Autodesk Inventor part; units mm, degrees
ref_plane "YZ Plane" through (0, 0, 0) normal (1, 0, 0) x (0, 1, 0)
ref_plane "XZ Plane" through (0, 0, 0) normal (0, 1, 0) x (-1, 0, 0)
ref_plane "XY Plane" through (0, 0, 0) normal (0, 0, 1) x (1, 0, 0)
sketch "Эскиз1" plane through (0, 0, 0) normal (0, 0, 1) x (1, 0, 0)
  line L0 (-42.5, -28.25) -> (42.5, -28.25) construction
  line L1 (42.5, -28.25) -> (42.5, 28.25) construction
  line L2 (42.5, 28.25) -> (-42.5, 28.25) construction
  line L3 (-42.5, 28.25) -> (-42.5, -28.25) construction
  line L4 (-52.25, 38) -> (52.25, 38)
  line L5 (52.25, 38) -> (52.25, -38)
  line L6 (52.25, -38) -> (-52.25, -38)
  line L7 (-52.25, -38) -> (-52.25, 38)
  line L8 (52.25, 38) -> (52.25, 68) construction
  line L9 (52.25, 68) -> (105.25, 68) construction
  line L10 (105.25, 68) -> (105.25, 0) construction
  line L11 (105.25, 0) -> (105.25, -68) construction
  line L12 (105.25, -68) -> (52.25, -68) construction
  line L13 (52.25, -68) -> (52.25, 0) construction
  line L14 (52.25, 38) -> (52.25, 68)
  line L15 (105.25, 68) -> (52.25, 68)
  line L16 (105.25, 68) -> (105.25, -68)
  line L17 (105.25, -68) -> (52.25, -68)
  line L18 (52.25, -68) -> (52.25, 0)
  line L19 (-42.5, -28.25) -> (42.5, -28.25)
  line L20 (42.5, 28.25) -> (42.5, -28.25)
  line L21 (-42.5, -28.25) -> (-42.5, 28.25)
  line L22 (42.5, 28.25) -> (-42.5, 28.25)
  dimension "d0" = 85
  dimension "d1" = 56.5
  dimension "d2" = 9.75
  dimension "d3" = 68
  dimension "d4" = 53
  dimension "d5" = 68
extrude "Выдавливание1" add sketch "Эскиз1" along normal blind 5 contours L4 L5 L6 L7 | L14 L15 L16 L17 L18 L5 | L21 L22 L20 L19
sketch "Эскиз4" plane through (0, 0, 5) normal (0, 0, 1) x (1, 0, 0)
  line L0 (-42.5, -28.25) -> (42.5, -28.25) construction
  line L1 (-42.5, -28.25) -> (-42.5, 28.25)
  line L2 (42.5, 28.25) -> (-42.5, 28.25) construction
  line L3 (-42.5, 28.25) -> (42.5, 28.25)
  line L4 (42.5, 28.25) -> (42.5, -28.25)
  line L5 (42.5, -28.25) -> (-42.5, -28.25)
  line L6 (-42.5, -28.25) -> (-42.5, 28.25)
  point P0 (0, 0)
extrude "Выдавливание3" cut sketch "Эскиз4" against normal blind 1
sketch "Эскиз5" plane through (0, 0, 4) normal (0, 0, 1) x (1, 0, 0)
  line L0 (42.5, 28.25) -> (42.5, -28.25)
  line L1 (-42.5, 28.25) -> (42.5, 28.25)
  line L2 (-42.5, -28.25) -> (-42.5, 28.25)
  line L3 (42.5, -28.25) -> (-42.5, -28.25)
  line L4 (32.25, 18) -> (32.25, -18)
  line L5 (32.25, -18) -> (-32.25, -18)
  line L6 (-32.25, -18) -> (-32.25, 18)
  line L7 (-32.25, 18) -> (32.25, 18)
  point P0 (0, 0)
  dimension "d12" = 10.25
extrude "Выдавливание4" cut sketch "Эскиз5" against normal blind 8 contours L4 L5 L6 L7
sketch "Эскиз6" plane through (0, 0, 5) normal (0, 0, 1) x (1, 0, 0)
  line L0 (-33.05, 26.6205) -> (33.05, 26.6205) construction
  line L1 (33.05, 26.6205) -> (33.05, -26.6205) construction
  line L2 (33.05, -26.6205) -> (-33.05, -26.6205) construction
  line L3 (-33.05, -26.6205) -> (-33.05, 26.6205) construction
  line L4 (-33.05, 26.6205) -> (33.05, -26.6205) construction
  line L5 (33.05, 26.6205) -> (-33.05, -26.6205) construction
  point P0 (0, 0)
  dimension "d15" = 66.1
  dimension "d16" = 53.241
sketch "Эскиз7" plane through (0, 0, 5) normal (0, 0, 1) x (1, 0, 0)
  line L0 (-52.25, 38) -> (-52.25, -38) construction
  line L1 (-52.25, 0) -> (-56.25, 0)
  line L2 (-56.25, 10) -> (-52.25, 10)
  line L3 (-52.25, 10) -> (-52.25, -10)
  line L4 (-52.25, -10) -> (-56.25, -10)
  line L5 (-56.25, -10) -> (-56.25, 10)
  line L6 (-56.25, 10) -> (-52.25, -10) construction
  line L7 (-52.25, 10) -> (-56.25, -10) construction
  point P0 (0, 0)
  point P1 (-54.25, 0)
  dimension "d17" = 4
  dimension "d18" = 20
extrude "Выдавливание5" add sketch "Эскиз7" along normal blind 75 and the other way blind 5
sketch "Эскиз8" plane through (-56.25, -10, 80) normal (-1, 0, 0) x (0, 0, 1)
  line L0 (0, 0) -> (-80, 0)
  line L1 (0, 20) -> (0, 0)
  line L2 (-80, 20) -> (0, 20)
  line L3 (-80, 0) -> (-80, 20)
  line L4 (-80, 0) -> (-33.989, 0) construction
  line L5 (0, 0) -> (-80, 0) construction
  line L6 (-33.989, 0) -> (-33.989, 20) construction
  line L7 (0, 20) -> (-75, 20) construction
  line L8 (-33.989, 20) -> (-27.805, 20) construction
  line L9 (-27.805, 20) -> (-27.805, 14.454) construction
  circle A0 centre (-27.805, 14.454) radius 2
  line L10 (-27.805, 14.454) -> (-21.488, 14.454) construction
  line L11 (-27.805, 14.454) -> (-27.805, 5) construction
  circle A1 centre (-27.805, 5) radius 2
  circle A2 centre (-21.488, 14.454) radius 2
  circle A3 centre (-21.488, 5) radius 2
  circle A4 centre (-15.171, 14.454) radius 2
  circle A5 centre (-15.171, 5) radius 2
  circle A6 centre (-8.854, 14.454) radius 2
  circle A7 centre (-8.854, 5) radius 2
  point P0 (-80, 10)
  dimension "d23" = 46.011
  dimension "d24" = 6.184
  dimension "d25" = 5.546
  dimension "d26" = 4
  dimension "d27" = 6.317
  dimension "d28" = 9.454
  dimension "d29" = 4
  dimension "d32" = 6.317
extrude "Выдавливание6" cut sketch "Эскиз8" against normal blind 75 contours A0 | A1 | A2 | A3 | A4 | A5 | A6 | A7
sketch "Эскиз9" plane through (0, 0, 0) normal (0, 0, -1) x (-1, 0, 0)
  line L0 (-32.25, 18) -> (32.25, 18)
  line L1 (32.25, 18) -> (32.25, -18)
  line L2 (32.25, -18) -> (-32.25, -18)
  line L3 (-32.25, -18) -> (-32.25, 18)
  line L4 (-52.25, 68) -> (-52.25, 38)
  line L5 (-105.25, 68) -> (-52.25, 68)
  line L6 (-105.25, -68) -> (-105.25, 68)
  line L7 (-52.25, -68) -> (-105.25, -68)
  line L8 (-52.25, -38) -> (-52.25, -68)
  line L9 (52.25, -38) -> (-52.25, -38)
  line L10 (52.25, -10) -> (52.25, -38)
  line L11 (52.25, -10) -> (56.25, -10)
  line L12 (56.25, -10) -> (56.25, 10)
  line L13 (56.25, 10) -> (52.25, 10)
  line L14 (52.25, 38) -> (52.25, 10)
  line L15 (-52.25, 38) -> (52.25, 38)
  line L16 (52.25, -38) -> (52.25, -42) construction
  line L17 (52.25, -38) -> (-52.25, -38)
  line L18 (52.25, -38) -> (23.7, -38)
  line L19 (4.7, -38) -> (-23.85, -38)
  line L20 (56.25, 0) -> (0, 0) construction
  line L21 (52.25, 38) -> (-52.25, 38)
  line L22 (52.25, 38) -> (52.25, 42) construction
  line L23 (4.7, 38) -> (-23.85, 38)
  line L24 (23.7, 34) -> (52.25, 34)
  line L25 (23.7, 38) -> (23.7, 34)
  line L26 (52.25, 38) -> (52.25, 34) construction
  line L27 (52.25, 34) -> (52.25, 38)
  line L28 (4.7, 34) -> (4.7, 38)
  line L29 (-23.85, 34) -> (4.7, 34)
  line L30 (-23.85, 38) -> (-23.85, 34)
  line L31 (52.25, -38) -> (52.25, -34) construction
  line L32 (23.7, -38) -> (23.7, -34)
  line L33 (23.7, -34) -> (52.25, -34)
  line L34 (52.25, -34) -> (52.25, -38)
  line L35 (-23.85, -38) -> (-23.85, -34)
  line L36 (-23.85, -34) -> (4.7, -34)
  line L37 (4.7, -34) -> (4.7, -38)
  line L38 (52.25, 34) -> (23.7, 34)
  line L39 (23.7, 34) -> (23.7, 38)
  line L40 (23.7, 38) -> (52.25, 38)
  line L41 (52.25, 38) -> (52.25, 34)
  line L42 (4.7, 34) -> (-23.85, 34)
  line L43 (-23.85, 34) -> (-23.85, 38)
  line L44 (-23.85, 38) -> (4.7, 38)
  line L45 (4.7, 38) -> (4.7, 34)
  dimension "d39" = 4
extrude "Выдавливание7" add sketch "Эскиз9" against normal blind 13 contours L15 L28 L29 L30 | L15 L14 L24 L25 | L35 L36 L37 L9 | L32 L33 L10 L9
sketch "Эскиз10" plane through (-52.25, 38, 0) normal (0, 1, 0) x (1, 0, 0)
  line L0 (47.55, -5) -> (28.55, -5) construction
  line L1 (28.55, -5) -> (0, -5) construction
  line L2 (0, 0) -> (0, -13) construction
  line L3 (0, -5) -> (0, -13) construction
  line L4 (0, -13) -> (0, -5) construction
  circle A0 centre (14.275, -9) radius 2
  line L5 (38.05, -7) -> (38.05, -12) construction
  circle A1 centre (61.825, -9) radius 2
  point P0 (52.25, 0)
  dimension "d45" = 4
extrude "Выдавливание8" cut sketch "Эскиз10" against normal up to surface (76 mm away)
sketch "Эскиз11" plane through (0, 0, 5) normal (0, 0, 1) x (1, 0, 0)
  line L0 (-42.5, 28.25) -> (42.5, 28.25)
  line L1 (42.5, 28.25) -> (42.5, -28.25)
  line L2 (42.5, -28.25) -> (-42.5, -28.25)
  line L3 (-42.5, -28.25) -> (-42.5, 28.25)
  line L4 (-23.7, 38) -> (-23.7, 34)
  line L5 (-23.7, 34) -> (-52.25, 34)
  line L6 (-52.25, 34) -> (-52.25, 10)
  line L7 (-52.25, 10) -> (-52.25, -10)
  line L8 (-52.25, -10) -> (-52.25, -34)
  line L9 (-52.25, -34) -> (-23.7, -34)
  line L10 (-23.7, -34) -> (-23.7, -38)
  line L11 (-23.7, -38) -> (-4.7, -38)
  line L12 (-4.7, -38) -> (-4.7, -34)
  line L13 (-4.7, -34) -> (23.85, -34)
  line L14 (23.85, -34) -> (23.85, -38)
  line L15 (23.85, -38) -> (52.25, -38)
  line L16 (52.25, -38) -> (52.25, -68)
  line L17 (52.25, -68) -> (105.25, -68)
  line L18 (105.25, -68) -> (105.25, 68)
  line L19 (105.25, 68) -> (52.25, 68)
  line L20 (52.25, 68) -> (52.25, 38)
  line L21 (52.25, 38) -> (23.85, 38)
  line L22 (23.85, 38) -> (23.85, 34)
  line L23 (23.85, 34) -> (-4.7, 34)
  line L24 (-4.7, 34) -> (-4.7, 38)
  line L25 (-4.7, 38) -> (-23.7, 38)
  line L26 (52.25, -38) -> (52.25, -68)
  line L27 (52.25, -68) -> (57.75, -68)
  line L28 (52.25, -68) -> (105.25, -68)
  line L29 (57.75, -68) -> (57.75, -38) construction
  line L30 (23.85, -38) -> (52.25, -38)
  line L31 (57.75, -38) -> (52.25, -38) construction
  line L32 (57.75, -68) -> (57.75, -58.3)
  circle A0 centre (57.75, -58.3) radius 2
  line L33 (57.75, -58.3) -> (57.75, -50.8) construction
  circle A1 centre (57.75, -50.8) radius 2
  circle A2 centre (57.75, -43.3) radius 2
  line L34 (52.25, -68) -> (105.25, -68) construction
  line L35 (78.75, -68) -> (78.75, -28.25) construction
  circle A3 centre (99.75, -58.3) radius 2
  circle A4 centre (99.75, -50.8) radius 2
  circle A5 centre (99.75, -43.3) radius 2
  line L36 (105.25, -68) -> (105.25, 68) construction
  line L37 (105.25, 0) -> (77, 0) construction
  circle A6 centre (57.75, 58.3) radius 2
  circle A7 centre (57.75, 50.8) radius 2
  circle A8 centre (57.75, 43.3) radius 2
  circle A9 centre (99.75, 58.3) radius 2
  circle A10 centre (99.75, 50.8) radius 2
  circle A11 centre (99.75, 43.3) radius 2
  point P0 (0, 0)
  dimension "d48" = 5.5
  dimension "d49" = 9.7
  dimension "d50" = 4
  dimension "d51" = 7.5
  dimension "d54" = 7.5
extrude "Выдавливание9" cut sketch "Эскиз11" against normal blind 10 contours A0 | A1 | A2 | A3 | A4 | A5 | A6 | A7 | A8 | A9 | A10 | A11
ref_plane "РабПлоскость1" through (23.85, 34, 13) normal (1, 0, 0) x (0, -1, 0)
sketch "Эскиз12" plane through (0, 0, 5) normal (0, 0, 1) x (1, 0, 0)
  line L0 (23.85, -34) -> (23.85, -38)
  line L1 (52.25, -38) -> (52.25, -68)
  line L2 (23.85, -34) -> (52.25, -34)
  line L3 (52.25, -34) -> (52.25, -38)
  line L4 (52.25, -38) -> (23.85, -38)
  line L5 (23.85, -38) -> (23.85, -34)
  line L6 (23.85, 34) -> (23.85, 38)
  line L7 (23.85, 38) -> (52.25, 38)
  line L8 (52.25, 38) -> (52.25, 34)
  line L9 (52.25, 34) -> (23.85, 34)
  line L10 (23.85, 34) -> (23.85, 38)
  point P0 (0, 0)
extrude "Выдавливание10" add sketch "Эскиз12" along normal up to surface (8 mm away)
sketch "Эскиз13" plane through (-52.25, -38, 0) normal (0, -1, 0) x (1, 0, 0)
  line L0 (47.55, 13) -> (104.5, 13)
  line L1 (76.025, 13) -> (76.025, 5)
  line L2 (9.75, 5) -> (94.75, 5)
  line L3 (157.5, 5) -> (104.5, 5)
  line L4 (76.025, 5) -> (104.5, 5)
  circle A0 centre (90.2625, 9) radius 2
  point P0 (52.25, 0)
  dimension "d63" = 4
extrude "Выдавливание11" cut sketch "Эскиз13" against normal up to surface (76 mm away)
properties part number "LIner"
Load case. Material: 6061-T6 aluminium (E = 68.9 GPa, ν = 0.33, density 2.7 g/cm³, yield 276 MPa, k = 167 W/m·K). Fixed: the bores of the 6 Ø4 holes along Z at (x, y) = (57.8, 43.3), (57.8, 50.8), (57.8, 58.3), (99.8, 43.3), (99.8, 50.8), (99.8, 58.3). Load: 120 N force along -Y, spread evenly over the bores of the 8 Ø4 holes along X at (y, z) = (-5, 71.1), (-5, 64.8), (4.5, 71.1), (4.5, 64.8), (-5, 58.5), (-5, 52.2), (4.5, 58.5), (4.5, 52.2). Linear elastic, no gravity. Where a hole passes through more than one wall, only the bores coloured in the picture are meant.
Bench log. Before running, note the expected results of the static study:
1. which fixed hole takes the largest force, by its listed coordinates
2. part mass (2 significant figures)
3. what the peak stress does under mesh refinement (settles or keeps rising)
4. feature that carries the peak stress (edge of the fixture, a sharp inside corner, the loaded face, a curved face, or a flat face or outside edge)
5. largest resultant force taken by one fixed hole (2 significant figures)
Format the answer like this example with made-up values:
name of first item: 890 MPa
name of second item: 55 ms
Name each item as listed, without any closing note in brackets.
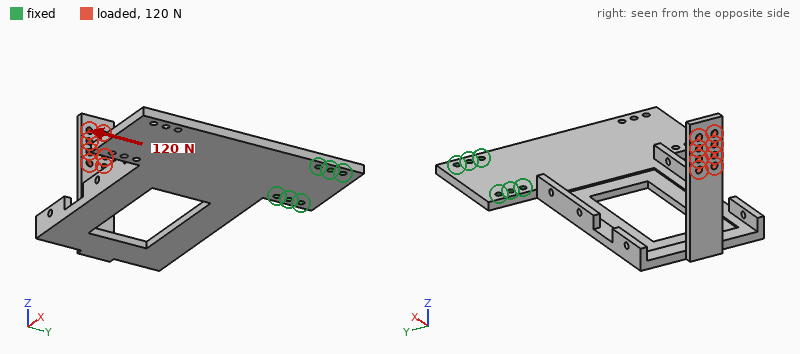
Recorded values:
which fixed hole takes the largest force, by its listed coordinates: (57.8, 43.3)
part mass: 190 g
what the peak stress does under mesh refinement: keeps rising
feature that carries the peak stress: edge of the fixture
largest resultant force taken by one fixed hole: 410 N
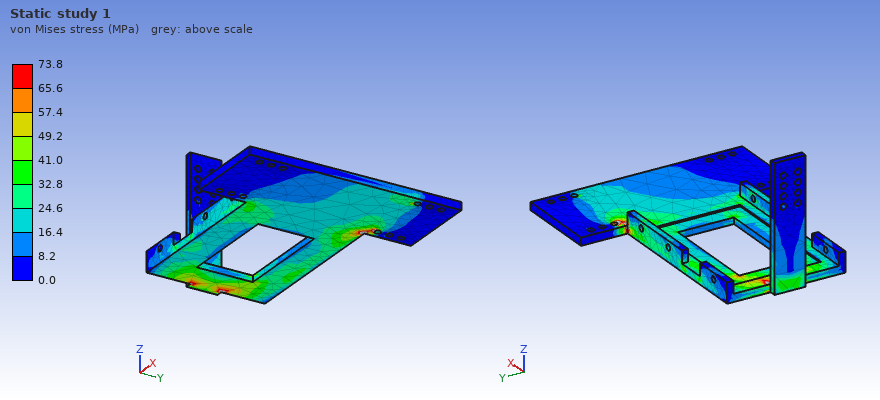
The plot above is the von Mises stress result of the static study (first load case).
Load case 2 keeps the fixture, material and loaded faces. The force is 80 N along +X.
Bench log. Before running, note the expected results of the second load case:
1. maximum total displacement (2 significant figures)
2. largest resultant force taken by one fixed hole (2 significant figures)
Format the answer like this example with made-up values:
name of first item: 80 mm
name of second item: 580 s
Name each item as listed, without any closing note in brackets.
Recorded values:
maximum total displacement: 2.4 mm
largest resultant force taken by one fixed hole: 150 N
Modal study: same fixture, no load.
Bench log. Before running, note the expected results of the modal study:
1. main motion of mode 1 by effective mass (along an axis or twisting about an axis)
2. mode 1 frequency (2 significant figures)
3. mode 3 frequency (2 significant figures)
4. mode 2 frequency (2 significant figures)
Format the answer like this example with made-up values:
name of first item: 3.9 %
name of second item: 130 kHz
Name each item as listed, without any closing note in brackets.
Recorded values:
main motion of mode 1 by effective mass: along Z
mode 1 frequency: 190 Hz
mode 3 frequency: 490 Hz
mode 2 frequency: 290 Hz
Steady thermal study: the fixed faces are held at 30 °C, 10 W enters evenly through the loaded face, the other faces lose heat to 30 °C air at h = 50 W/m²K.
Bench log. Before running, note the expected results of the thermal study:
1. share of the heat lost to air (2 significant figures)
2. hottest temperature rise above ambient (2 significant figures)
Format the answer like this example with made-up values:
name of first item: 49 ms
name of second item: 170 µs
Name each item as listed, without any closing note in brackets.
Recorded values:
share of the heat lost to air: 88 %
hottest temperature rise above ambient: 41 K
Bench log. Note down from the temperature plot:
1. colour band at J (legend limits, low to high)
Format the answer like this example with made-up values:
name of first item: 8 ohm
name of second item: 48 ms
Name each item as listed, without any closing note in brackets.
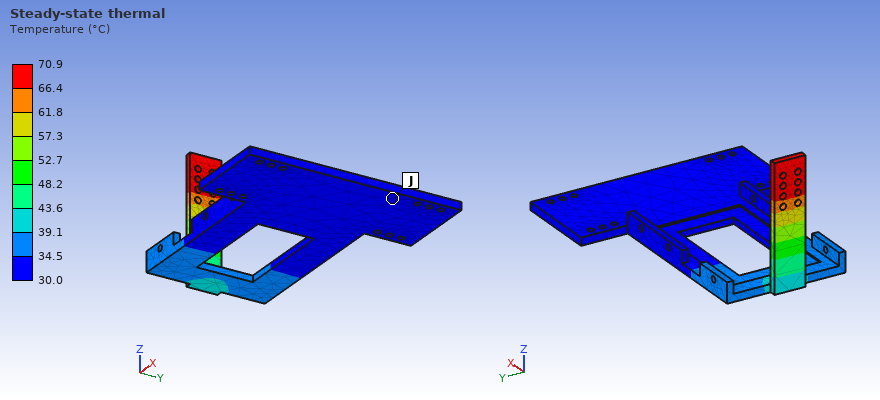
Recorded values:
colour band at J: 30.0 to 34.5 °C
